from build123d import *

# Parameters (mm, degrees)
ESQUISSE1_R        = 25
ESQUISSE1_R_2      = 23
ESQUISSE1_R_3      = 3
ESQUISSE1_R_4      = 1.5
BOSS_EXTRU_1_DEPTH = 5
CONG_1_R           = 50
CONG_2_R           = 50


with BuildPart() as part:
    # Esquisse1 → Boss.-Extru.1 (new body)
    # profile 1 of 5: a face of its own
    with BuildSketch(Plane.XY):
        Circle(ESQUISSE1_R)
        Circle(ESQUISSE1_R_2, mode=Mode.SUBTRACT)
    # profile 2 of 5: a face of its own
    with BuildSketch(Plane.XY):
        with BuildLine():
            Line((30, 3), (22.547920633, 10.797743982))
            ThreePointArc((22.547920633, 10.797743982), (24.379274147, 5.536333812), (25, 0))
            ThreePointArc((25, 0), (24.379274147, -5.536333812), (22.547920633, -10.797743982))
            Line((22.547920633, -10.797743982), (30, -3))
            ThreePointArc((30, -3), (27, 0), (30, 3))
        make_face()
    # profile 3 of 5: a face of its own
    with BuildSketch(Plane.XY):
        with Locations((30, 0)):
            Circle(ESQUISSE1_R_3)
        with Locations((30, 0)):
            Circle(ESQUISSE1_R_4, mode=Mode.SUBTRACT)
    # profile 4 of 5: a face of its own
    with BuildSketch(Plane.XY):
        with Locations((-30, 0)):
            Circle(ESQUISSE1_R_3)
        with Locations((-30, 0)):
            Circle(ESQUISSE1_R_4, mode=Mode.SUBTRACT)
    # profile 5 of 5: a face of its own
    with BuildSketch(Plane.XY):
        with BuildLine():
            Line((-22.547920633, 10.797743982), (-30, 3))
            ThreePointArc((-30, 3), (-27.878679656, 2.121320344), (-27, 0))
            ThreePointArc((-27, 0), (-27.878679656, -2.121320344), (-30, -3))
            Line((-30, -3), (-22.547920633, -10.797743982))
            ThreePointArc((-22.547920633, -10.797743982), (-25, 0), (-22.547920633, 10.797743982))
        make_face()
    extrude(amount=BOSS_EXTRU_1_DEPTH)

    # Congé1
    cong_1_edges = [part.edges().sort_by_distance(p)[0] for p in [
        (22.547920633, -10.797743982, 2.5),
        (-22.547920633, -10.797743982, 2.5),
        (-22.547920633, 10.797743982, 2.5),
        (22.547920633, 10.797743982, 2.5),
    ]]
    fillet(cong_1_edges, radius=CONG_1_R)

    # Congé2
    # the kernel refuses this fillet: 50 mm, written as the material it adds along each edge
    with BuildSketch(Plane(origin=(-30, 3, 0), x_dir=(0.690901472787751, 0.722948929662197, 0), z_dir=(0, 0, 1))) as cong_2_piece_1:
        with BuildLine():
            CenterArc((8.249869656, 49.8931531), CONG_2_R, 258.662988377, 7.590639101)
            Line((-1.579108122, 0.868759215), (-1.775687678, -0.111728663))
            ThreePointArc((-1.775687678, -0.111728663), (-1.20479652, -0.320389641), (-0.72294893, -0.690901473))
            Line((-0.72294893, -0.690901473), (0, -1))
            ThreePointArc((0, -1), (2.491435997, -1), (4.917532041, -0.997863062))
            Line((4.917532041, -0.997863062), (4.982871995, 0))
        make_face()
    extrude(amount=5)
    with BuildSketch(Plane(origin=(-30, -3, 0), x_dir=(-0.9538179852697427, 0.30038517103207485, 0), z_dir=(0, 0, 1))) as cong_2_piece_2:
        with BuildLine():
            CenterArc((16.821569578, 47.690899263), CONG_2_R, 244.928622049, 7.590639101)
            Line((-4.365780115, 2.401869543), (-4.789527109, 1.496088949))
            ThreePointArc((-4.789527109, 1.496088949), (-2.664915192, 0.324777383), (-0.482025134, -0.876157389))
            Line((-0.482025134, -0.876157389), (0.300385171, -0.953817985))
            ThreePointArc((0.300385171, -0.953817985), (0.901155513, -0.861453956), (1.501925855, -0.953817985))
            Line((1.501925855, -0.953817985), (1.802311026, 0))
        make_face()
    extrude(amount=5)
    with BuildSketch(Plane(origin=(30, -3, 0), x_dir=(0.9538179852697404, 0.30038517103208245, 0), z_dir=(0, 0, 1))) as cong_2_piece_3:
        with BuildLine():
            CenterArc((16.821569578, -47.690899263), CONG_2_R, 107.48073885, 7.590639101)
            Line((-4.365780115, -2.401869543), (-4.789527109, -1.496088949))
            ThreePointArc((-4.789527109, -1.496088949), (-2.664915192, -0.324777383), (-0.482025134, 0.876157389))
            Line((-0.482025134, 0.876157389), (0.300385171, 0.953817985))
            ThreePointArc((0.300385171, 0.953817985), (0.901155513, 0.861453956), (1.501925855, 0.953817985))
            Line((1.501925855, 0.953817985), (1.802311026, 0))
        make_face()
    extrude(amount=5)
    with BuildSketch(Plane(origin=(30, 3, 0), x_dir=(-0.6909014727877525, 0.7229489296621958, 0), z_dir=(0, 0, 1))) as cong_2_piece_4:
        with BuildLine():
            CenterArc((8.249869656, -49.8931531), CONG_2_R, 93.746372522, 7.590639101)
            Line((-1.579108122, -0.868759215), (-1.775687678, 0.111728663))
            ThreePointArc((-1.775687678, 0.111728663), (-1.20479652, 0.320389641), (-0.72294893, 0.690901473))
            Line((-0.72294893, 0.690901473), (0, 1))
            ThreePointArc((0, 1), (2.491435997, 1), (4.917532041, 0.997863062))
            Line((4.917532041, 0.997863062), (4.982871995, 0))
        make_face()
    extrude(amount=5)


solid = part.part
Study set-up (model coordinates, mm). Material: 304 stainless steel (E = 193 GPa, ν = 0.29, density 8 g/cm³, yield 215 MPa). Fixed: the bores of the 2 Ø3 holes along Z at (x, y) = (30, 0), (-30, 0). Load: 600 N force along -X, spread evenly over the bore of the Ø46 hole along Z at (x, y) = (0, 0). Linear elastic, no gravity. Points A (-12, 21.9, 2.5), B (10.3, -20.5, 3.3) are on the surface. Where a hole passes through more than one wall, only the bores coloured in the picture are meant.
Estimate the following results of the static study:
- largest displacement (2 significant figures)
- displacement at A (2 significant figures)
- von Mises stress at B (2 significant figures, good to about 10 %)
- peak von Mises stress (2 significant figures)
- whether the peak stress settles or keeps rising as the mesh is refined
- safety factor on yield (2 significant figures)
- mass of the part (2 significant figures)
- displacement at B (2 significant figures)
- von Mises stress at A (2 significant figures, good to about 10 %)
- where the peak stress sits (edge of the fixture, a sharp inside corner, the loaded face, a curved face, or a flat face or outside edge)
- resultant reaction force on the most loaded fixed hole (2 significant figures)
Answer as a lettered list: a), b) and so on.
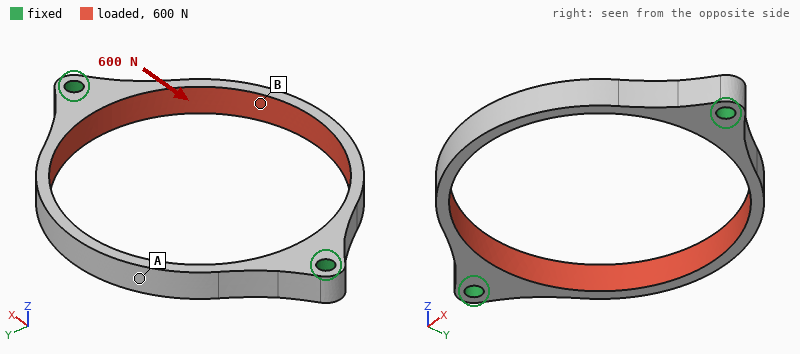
a) 34 µm
b) 33 µm
c) 76 MPa
d) 79 MPa
e) settles
f) 2.7
g) 18 g
h) 33 µm
i) 62 MPa
j) a curved face
k) 300 N
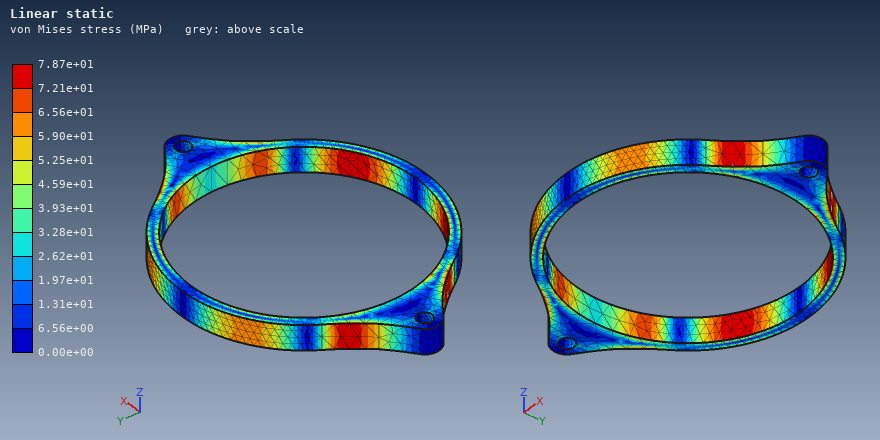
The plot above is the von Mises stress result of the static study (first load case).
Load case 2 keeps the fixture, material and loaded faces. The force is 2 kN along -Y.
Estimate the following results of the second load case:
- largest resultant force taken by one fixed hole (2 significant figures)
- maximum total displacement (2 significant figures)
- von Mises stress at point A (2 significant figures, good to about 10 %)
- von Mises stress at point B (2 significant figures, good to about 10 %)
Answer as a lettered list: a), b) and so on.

a) 1.0 kN
b) 16 µm
c) 19 MPa
d) 41 MPa
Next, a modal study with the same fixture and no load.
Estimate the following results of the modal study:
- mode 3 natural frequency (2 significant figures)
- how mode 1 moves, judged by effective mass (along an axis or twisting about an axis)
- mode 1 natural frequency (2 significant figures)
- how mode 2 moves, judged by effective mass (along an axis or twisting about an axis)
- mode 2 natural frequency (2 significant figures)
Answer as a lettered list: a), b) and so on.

a) 5800 Hz
b) twisting about X
c) 4000 Hz
d) along Z
e) 4300 Hz
